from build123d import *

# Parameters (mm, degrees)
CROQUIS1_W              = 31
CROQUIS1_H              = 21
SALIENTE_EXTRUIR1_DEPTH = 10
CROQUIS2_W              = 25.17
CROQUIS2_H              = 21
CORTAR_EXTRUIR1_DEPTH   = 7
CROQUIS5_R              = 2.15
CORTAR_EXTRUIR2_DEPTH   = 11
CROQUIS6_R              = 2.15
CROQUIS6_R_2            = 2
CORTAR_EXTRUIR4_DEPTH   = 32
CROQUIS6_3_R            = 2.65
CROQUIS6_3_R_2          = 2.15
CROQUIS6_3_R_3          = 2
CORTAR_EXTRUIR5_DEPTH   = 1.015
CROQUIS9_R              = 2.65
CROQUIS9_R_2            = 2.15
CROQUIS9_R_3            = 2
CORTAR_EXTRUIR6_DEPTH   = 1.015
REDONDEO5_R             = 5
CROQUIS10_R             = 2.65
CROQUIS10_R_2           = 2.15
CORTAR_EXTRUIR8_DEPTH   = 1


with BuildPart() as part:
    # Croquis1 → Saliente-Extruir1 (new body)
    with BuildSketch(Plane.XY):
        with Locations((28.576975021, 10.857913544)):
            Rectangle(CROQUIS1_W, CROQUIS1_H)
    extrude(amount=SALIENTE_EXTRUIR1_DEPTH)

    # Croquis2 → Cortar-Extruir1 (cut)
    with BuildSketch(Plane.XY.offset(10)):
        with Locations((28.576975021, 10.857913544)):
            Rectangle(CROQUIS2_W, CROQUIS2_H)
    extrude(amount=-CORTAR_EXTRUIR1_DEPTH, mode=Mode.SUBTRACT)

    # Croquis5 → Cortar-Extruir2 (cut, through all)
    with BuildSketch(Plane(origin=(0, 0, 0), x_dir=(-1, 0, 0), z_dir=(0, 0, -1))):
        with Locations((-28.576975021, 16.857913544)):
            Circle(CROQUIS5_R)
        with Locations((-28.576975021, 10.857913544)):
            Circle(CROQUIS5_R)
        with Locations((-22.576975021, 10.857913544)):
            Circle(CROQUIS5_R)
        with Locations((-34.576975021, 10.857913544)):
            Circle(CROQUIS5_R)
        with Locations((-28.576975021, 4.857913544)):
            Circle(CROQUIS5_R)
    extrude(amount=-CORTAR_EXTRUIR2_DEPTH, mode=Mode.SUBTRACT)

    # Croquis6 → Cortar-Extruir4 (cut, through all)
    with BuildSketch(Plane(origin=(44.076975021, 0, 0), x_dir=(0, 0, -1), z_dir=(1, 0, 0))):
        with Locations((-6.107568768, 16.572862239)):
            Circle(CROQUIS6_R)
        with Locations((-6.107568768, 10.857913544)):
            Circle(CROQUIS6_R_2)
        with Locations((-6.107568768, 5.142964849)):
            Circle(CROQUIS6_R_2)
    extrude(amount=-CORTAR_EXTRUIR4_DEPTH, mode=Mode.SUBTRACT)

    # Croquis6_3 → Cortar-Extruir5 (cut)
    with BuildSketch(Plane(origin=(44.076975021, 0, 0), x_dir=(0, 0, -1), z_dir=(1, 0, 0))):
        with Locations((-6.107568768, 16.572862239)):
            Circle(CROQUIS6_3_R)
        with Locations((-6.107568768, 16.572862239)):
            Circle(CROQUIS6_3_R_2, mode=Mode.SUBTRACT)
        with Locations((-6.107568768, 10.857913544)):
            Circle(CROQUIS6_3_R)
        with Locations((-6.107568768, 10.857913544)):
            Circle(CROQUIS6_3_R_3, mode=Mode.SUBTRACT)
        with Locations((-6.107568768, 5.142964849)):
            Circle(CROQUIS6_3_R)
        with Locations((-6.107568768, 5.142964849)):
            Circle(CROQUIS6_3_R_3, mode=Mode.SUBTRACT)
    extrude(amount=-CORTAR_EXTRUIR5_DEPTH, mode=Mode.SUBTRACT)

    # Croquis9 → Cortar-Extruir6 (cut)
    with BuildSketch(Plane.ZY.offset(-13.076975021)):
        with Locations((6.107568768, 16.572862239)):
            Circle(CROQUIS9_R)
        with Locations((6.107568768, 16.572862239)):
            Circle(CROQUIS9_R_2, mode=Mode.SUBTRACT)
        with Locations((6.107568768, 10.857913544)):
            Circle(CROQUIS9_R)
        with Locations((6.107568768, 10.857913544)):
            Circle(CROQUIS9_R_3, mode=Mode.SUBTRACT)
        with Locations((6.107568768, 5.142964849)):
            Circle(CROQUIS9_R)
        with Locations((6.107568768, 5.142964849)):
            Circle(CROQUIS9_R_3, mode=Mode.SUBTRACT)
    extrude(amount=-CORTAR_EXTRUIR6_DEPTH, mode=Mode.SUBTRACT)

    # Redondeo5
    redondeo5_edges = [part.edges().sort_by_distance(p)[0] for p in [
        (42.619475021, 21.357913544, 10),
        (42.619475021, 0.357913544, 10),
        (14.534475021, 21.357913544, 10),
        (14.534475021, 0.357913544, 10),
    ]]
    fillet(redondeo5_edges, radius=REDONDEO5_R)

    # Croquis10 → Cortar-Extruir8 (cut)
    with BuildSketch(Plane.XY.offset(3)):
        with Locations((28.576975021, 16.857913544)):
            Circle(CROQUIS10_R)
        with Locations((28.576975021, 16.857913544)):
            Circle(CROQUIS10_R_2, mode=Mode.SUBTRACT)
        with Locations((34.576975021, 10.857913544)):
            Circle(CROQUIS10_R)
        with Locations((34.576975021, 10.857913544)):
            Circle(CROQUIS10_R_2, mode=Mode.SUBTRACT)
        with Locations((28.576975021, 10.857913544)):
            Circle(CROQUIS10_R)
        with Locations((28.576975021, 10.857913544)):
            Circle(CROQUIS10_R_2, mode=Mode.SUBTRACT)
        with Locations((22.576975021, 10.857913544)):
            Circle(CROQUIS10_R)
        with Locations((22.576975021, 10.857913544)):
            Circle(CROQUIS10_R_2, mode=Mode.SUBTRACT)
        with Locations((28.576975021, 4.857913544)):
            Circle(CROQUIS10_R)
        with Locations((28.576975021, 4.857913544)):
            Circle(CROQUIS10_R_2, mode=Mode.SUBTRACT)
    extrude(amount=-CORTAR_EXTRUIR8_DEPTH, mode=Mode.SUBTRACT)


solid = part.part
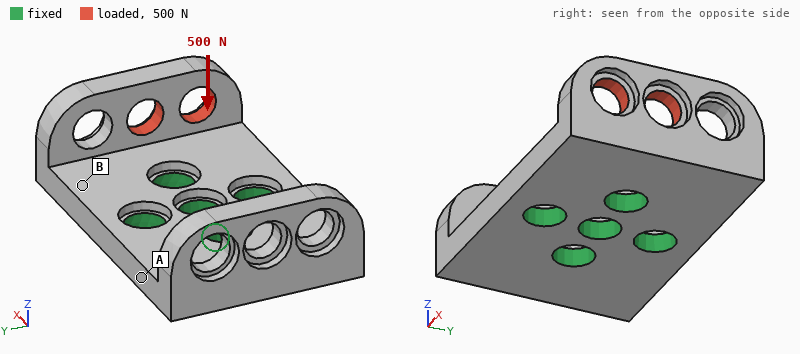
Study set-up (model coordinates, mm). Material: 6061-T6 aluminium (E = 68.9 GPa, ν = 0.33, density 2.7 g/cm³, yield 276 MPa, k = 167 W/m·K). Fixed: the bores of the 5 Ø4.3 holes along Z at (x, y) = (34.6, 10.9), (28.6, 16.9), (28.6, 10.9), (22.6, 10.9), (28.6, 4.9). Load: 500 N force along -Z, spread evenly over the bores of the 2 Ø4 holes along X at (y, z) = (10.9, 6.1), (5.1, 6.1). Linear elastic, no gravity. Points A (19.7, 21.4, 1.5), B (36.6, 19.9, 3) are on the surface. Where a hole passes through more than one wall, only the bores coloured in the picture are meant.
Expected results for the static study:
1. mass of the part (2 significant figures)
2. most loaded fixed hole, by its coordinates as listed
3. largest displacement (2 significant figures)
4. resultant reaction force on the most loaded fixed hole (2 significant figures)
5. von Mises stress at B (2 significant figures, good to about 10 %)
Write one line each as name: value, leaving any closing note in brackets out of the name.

mass of the part: 6.0 g
most loaded fixed hole, by its coordinates as listed: (34.6, 10.9)
largest displacement: 76 µm
resultant reaction force on the most loaded fixed hole: 720 N
von Mises stress at B: 43 MPa
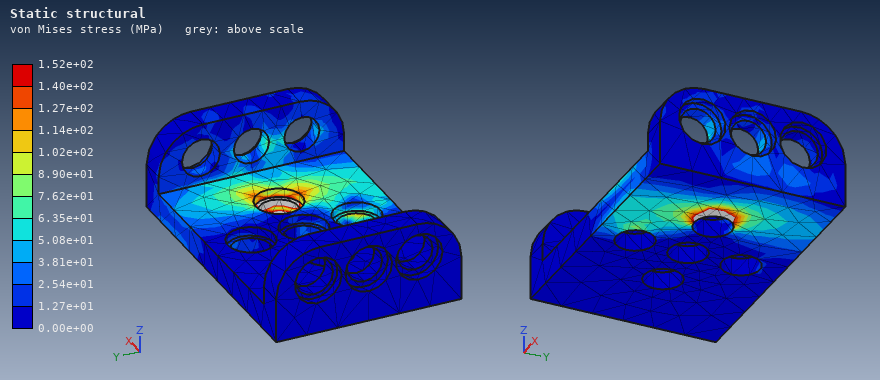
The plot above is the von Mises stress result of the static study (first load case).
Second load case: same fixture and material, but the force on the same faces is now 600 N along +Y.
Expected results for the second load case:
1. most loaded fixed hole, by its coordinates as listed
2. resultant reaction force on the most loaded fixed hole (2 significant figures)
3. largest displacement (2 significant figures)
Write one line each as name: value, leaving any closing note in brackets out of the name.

most loaded fixed hole, by its coordinates as listed: (34.6, 10.9)
resultant reaction force on the most loaded fixed hole: 540 N
largest displacement: 57 µm
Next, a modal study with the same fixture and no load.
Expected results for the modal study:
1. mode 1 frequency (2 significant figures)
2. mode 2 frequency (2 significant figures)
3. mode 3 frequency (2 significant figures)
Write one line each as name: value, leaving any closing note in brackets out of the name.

mode 1 frequency: 13 kHz
mode 2 frequency: 13 kHz
mode 3 frequency: 14 kHz
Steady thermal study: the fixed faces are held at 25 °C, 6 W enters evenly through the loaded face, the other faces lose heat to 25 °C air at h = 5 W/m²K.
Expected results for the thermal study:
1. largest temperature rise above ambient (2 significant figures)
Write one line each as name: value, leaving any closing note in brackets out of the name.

largest temperature rise above ambient: 12 K
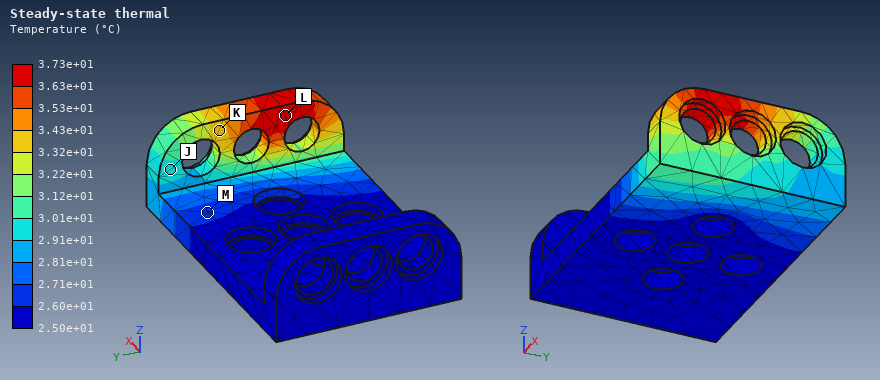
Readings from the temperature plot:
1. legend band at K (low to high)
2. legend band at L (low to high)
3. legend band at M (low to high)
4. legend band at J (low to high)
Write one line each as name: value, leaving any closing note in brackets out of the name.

legend band at K: 3.32e+01 to 3.43e+01 °C
legend band at L: 3.63e+01 to 3.73e+01 °C
legend band at M: 2.60e+01 to 2.71e+01 °C
legend band at J: 2.91e+01 to 3.01e+01 °C
